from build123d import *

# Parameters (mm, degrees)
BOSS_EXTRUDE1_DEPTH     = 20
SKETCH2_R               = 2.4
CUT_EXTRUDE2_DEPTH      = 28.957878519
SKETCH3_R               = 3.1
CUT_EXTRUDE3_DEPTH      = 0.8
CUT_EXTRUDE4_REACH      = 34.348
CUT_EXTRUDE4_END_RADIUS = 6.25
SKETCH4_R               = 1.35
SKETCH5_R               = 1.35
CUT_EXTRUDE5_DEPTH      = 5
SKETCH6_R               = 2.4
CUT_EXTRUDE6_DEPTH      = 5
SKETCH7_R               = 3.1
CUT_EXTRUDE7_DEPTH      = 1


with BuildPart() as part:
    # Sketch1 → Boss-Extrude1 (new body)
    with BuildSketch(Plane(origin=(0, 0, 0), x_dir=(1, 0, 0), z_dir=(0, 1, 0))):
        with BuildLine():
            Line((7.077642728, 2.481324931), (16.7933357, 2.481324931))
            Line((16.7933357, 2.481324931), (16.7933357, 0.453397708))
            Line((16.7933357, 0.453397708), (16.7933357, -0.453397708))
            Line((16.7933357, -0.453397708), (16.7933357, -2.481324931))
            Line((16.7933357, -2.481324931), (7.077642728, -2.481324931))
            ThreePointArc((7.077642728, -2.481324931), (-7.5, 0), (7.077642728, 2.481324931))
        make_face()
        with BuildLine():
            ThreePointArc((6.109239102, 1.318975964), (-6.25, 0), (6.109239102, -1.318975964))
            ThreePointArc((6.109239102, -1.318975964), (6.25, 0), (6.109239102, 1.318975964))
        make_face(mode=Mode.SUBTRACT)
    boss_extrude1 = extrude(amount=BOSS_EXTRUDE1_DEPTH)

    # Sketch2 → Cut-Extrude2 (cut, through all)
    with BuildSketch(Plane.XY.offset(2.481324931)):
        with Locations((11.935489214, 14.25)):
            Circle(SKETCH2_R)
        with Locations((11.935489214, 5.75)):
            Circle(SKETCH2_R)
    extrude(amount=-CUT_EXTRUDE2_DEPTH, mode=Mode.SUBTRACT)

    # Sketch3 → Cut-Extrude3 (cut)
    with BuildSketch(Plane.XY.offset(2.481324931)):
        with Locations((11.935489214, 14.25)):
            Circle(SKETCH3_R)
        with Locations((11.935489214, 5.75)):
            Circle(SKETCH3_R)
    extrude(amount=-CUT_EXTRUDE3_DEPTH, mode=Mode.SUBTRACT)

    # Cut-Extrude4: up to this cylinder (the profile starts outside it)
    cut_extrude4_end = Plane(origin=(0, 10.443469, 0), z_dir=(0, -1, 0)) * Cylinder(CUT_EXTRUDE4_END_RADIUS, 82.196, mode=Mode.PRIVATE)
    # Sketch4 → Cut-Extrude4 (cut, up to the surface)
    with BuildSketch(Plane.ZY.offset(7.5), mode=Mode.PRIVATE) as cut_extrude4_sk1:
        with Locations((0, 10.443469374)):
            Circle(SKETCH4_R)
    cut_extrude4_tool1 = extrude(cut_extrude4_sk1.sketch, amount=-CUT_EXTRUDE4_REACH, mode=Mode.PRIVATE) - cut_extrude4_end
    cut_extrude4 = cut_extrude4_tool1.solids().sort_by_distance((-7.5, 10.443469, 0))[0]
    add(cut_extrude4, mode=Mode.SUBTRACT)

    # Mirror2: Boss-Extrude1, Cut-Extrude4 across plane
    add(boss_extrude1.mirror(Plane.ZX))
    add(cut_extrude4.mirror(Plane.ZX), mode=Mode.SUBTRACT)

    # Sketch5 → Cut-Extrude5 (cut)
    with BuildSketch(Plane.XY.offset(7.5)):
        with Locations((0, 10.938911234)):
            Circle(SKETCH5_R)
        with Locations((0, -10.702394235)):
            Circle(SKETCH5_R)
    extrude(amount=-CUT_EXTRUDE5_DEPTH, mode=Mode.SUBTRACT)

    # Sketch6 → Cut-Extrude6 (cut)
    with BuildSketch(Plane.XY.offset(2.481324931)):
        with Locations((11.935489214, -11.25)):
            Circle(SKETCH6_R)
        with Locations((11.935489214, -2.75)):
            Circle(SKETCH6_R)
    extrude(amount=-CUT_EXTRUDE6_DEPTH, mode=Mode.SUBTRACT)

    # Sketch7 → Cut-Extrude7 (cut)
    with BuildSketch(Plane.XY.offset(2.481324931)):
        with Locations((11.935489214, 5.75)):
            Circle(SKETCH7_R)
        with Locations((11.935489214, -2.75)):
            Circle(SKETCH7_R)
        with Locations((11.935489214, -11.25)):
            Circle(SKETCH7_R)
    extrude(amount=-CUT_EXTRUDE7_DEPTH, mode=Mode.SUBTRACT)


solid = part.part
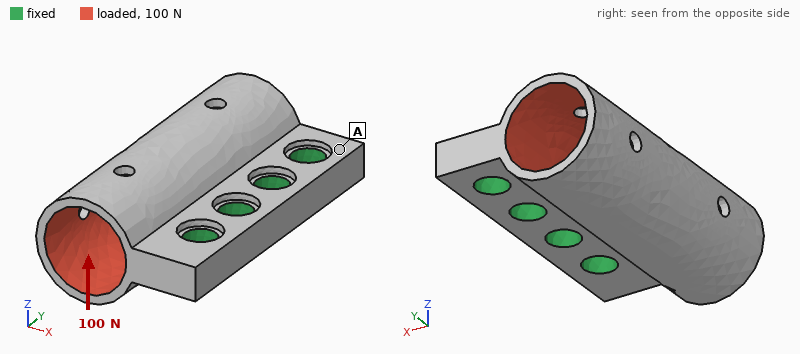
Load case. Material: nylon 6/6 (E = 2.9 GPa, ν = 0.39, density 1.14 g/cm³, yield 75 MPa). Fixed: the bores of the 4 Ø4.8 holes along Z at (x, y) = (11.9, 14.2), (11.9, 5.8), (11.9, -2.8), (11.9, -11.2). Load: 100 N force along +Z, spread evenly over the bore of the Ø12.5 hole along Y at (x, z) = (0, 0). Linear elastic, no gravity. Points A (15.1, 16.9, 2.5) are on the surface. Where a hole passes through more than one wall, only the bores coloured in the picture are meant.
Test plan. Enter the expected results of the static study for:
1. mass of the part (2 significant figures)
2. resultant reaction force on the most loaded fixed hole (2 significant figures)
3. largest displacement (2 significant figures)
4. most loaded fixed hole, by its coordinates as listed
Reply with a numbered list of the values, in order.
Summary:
1. 4.1 g
2. 32 N
3. 0.56 mm
4. (11.9, -11.2)
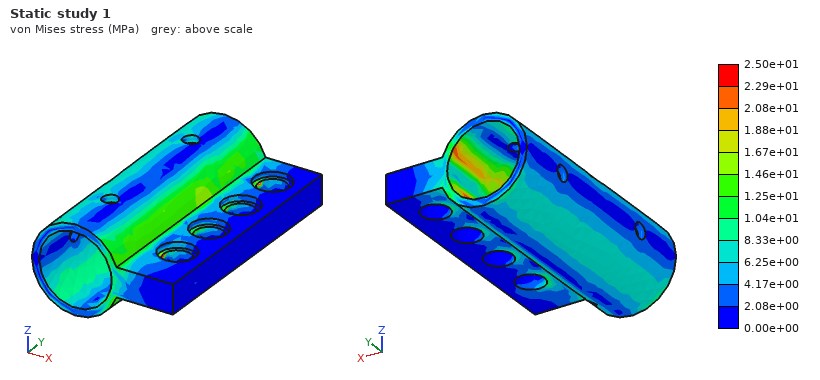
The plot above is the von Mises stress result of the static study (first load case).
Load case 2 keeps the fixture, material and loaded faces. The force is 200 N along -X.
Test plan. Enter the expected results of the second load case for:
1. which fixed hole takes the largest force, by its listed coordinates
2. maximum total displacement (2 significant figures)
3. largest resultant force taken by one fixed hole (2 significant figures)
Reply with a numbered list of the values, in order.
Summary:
1. (11.9, -11.2)
2. 0.15 mm
3. 70 N
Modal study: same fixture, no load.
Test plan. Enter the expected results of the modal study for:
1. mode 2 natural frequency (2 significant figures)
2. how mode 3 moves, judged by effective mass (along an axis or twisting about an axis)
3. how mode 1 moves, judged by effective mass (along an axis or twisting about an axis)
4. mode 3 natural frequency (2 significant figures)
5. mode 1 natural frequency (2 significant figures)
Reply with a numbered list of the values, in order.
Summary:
1. 3800 Hz
2. along X
3. along Z
4. 4100 Hz
5. 1500 Hz
